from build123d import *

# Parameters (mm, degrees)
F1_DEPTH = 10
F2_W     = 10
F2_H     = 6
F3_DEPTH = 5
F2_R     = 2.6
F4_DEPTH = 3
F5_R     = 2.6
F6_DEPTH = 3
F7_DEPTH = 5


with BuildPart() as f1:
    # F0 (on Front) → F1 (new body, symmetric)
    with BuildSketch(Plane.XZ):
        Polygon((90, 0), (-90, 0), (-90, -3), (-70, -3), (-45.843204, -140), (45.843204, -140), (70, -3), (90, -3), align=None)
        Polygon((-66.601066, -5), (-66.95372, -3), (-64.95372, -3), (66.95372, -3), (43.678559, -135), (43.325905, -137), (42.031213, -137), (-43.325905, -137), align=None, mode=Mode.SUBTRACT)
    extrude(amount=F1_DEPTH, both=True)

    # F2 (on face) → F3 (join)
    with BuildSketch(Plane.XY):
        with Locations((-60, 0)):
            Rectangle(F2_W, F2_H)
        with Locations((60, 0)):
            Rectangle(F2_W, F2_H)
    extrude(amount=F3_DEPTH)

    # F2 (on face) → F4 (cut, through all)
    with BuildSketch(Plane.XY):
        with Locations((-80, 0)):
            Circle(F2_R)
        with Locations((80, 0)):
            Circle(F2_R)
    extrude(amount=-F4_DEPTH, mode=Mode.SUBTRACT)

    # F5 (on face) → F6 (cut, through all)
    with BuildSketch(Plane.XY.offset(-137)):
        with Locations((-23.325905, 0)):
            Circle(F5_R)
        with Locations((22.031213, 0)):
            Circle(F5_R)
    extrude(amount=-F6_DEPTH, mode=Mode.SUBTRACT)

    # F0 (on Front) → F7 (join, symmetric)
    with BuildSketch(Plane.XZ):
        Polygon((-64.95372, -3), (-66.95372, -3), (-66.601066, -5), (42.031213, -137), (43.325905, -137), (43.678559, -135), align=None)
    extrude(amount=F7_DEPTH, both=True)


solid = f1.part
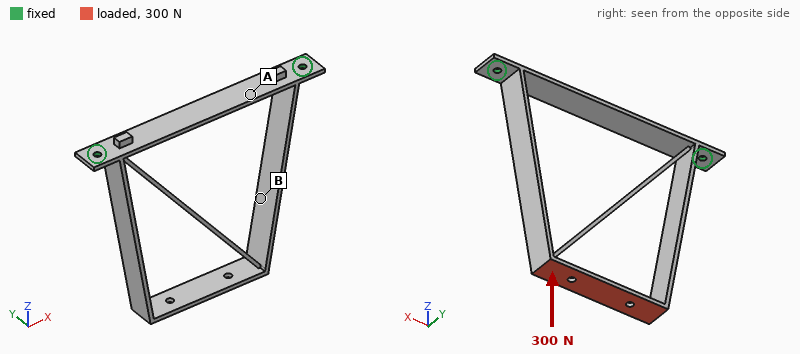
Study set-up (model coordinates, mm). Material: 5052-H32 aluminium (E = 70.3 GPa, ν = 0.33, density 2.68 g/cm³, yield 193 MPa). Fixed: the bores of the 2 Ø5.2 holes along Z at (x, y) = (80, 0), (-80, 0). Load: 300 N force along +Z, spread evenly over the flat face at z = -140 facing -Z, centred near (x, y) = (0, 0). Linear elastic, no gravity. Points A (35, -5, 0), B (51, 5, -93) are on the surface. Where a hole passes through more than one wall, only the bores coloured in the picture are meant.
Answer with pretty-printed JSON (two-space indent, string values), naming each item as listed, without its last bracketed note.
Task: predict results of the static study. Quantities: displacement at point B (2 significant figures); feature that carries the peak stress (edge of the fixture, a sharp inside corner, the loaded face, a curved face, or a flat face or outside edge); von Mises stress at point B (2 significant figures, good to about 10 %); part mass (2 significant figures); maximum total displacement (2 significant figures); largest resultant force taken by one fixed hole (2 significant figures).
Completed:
{
  "displacement at point B": "0.25 mm",
  "feature that carries the peak stress": "the loaded face",
  "von Mises stress at point B": "22 MPa",
  "part mass": "100 g",
  "maximum total displacement": "0.46 mm",
  "largest resultant force taken by one fixed hole": "150 N"
}
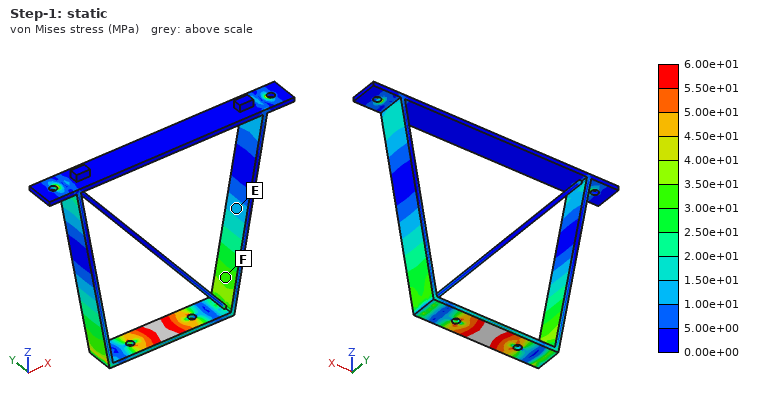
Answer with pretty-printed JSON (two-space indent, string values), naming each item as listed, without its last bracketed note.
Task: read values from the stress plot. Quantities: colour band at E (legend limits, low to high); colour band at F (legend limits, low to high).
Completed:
{
  "colour band at E": "1.00e+01 to 1.50e+01 MPa",
  "colour band at F": "3.00e+01 to 3.50e+01 MPa"
}
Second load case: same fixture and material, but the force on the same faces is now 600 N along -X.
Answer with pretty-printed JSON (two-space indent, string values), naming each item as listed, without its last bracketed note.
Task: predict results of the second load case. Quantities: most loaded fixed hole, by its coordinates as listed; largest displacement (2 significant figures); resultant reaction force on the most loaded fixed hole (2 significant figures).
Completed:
{
  "most loaded fixed hole, by its coordinates as listed": "(-80, 0)",
  "largest displacement": "0.22 mm",
  "resultant reaction force on the most loaded fixed hole": "740 N"
}
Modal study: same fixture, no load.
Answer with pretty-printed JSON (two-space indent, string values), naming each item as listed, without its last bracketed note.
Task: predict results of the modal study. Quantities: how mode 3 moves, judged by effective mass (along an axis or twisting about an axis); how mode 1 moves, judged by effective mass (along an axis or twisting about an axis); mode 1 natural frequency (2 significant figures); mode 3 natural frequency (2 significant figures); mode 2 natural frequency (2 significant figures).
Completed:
{
  "how mode 3 moves, judged by effective mass": "twisting about Z",
  "how mode 1 moves, judged by effective mass": "along Y",
  "mode 1 natural frequency": "220 Hz",
  "mode 3 natural frequency": "490 Hz",
  "mode 2 natural frequency": "420 Hz"
}
